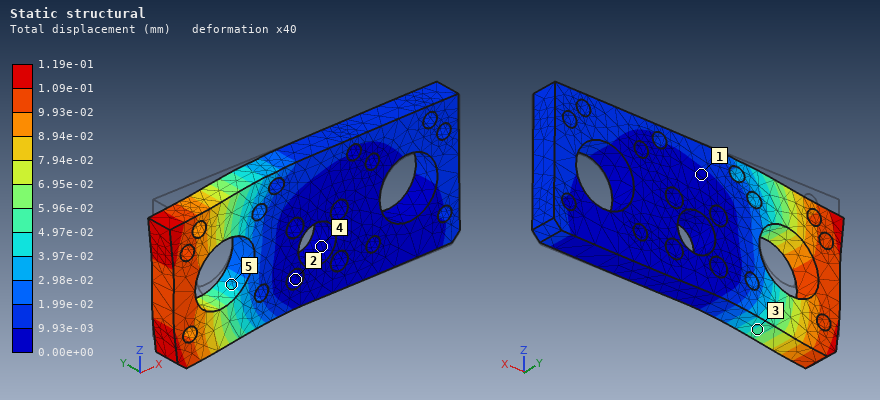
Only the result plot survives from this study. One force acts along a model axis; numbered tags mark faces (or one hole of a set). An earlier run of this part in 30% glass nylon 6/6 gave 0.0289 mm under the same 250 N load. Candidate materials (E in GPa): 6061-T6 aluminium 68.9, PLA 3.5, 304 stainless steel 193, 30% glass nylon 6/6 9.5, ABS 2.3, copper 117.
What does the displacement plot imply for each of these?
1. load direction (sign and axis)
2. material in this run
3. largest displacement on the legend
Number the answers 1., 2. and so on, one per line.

1. -Z
2. ABS
3. 1.19e-01 mm
